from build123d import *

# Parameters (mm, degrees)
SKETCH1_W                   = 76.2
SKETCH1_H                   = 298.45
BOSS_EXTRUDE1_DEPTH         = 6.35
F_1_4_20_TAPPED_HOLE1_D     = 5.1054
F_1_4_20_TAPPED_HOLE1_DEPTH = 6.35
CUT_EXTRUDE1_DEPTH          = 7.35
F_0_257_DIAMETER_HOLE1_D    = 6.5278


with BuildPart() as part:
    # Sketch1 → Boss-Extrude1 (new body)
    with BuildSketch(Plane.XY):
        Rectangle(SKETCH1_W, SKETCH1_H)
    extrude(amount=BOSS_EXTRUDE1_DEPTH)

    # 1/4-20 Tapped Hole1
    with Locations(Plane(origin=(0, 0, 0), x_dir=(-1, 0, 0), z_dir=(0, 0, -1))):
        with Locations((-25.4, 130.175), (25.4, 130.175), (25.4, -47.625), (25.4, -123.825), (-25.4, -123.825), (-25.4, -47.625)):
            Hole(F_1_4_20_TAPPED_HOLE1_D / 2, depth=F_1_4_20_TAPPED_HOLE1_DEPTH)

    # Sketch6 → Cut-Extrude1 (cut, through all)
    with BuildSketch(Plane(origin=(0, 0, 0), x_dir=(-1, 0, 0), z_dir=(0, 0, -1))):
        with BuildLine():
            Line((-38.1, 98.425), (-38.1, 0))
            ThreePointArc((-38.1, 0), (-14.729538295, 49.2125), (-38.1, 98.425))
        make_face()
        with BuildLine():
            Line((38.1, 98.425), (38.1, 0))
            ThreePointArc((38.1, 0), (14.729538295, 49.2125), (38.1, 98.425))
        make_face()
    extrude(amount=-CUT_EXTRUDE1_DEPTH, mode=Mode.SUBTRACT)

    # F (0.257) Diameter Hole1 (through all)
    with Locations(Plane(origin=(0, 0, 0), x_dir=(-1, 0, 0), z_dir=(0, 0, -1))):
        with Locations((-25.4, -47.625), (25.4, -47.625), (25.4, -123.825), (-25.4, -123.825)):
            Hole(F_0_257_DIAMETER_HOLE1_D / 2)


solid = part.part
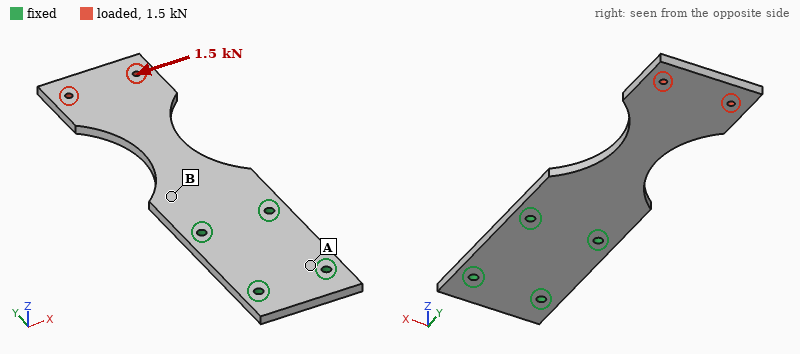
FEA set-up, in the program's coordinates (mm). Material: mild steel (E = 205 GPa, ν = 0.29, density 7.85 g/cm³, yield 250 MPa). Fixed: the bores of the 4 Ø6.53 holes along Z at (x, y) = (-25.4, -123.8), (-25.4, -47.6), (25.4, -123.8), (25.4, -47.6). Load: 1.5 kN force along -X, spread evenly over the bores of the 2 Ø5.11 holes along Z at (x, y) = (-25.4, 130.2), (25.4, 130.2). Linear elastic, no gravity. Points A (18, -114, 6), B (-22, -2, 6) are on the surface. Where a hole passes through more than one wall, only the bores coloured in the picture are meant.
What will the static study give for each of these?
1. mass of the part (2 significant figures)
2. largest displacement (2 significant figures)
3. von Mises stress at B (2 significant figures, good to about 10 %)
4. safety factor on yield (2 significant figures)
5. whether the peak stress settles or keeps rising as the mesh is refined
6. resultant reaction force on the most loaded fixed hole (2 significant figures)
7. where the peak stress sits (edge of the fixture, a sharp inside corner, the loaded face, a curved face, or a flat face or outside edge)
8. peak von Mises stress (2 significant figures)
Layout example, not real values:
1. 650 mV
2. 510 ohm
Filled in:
1. 970 g
2. 0.31 mm
3. 34 MPa
4. 1.7
5. settles
6. 4.5 kN
7. a curved face
8. 150 MPa
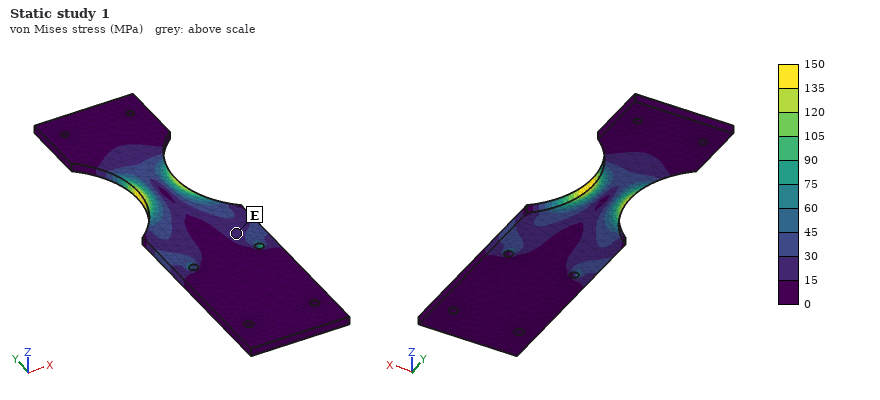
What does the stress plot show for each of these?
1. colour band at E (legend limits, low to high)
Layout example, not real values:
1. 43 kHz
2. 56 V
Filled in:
1. 15 to 30 MPa
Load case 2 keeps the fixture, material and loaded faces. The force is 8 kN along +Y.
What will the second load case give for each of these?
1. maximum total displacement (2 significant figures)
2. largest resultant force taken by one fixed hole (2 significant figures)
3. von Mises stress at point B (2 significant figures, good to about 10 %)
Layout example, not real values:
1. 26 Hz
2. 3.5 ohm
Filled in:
1. 26 µm
2. 3.6 kN
3. 19 MPa
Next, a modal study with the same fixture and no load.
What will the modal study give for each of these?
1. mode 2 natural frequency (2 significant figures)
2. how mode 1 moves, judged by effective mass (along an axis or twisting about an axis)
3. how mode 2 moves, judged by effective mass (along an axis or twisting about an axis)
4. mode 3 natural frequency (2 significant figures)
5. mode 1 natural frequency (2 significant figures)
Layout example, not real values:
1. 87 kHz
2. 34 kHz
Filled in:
1. 660 Hz
2. along Z
3. twisting about Y
4. 840 Hz
5. 120 Hz
